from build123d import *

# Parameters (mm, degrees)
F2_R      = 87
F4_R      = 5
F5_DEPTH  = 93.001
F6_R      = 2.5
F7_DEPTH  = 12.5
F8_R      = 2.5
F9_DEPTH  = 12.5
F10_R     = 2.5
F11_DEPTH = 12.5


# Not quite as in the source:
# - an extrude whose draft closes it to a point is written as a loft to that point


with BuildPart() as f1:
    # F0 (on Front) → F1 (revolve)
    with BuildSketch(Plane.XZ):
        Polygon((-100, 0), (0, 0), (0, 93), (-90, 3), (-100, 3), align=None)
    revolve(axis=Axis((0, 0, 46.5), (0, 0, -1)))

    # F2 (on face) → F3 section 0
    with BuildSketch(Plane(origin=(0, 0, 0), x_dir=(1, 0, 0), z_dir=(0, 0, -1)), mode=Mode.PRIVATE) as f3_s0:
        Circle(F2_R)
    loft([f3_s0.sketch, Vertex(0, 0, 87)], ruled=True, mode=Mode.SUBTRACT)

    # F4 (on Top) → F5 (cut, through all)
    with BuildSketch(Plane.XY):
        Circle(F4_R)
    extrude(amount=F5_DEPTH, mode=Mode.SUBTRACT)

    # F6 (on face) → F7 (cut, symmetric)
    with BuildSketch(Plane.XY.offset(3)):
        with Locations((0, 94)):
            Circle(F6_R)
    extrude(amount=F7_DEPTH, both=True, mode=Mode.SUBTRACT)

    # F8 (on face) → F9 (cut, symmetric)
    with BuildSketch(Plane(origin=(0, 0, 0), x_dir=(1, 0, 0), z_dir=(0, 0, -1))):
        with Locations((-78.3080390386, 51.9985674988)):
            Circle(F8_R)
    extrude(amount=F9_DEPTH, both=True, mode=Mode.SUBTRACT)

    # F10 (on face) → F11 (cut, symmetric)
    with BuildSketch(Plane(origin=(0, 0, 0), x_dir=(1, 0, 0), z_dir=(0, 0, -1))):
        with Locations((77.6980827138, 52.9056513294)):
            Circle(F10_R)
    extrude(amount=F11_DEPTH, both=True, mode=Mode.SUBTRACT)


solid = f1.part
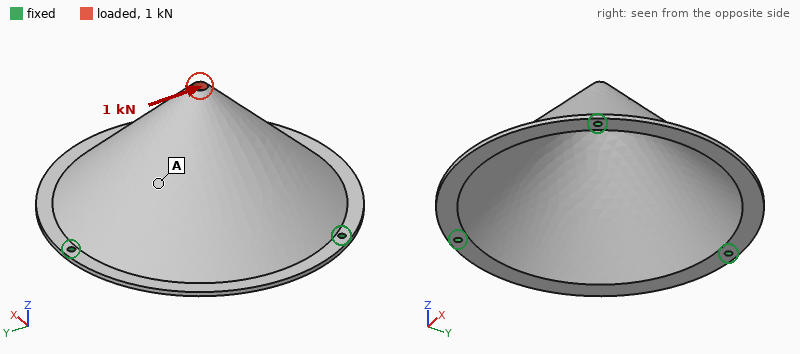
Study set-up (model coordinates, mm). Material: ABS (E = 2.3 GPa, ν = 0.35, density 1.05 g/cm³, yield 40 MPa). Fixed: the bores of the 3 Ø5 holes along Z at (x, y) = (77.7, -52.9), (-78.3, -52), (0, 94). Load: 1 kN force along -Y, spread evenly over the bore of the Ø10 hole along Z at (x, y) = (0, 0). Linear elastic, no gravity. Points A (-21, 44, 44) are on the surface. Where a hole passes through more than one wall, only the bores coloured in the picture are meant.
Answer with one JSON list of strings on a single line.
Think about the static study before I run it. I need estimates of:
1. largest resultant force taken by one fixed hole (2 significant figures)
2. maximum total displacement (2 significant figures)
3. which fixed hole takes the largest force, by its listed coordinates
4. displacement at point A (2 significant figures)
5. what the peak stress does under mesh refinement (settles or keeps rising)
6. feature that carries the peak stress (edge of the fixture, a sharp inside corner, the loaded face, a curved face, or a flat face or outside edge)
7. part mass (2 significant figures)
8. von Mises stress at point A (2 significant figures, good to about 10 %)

["880 N", "0.66 mm", "(0, 94)", "0.30 mm", "keeps rising", "edge of the fixture", "180 g", "3.1 MPa"]
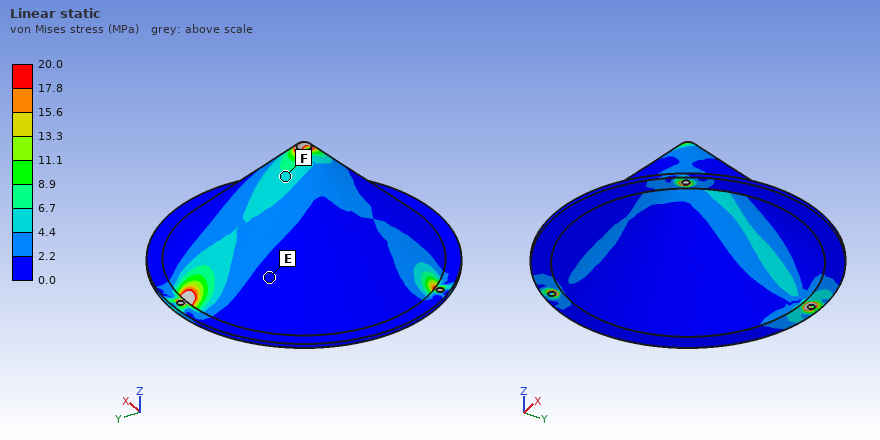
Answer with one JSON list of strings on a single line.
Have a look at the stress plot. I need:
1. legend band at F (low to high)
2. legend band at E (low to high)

["4.4 to 6.7 MPa", "0.0 to 2.2 MPa"]
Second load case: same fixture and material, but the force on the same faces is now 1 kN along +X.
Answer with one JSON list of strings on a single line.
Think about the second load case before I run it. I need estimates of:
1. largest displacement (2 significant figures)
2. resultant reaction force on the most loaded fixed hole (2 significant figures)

["0.75 mm", "820 N"]
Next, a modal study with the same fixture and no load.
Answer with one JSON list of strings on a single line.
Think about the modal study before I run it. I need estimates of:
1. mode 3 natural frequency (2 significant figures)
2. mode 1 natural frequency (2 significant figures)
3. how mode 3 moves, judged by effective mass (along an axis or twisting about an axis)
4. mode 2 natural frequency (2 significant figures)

["720 Hz", "620 Hz", "twisting about Y", "630 Hz"]
